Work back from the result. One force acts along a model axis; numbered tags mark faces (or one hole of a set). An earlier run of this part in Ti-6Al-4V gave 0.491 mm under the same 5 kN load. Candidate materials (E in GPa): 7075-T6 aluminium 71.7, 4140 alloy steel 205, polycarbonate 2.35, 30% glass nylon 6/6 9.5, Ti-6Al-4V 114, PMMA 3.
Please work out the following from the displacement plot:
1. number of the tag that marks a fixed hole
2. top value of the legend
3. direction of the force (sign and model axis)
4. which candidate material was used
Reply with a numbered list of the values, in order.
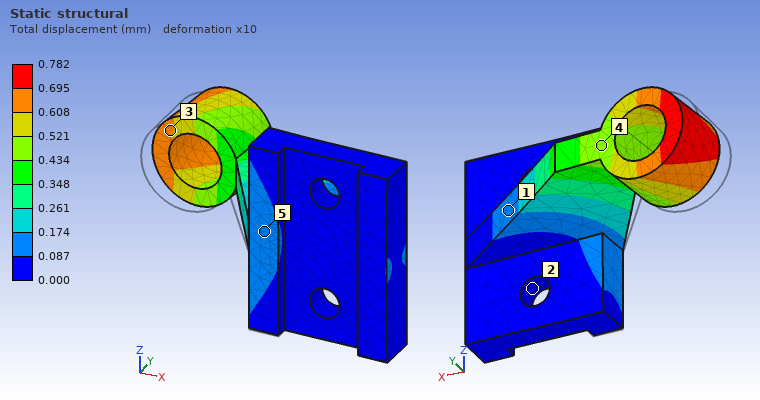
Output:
1. 2
2. 0.782 mm
3. +Y
4. 7075-T6 aluminium
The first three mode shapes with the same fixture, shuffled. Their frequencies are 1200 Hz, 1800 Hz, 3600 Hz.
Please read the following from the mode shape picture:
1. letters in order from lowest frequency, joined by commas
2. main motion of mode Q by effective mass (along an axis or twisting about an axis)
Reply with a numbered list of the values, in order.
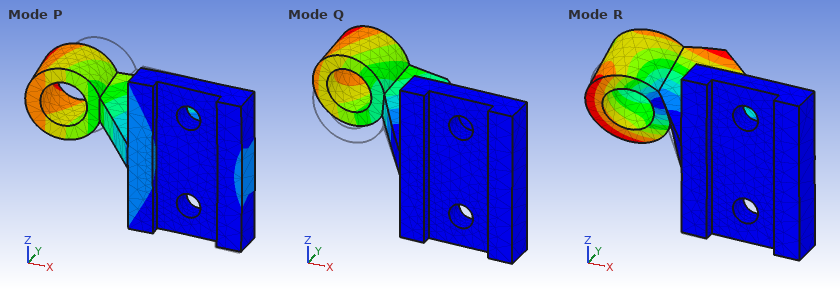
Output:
1. Q, P, R
2. along Z
